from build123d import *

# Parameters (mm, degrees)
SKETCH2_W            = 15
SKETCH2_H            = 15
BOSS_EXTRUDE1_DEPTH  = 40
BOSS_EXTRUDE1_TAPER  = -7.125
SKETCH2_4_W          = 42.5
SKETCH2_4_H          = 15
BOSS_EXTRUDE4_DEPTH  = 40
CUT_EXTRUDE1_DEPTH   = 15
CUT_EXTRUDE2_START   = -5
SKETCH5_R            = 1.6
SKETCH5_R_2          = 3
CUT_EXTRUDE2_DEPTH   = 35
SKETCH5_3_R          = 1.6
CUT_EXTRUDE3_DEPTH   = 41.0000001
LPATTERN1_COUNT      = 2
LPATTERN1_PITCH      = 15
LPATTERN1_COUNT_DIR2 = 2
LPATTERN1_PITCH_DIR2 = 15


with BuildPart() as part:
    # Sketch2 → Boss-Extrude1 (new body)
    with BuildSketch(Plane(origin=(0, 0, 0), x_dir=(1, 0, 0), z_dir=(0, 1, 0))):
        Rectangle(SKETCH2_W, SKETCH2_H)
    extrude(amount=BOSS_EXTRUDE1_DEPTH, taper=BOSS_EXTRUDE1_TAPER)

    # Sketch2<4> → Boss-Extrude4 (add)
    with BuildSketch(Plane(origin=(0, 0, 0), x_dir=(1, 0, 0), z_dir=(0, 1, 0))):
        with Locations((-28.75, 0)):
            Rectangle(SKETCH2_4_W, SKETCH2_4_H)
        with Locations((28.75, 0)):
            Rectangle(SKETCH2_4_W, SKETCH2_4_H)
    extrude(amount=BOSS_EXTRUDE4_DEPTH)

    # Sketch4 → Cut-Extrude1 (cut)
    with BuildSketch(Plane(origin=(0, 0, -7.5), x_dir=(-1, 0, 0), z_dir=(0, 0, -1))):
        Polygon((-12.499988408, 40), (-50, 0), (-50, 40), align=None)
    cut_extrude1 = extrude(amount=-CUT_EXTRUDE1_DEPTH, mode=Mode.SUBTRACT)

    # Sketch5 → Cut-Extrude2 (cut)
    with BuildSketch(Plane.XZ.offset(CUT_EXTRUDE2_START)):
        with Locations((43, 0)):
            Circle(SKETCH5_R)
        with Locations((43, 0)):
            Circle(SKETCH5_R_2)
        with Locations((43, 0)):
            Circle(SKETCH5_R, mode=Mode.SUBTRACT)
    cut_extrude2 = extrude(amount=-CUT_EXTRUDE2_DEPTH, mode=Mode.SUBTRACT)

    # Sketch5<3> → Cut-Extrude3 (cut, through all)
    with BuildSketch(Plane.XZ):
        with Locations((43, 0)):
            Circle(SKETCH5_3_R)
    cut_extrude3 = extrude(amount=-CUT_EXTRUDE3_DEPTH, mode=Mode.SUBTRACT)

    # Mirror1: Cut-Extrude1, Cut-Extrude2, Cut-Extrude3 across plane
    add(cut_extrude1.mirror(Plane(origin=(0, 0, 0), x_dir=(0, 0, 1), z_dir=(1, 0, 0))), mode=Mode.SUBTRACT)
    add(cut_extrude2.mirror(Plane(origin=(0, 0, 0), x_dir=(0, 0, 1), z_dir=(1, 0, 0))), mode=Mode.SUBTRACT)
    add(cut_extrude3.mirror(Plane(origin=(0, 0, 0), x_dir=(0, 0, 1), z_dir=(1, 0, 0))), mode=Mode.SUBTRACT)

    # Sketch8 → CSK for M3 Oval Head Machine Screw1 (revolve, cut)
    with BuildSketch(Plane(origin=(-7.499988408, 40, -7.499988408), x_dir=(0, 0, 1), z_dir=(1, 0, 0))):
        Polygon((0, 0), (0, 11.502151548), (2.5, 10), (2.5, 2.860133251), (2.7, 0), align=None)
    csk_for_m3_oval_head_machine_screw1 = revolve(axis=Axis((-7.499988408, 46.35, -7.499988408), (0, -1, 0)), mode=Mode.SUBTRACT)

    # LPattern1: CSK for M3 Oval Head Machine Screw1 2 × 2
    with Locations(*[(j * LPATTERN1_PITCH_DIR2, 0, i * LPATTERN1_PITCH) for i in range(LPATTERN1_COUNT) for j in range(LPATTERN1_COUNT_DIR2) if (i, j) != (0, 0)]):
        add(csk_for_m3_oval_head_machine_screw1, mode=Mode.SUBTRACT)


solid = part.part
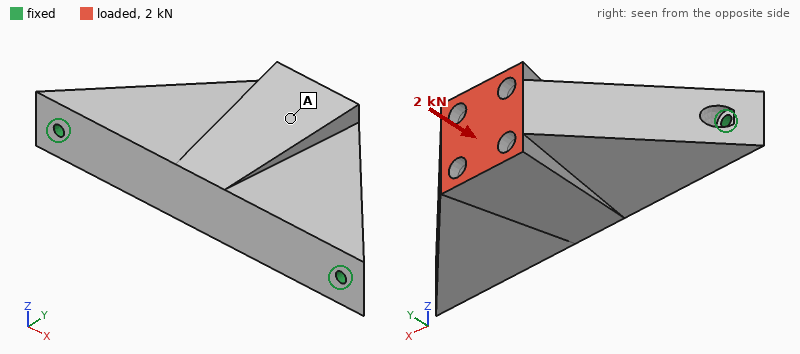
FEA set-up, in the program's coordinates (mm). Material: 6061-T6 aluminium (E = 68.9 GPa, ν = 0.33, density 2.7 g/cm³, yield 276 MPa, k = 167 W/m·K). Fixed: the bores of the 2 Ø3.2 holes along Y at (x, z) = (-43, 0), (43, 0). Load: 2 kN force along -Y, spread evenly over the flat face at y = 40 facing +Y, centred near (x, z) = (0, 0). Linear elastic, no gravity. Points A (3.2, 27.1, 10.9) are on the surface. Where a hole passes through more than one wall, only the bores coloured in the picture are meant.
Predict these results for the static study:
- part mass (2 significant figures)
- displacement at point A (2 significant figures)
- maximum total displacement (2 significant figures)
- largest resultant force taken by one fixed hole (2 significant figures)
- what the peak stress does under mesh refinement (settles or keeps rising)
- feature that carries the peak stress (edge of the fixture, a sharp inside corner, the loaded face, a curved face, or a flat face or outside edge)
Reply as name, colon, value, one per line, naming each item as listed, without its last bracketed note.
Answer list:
part mass: 110 g
displacement at point A: 11 µm
maximum total displacement: 12 µm
largest resultant force taken by one fixed hole: 1.3 kN
what the peak stress does under mesh refinement: keeps rising
feature that carries the peak stress: edge of the fixture
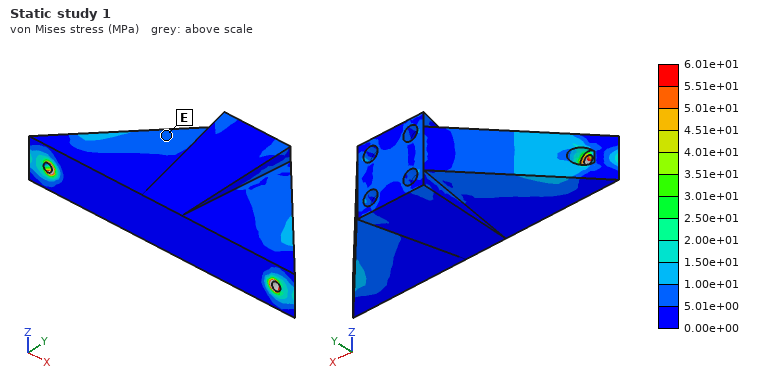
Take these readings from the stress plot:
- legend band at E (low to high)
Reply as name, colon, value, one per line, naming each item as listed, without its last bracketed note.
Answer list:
legend band at E: 5.01e+00 to 1.00e+01 MPa
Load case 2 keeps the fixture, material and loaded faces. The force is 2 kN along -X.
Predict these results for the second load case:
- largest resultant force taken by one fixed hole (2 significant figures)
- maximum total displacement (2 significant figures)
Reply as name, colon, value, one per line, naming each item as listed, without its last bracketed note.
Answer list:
largest resultant force taken by one fixed hole: 1.3 kN
maximum total displacement: 11 µm
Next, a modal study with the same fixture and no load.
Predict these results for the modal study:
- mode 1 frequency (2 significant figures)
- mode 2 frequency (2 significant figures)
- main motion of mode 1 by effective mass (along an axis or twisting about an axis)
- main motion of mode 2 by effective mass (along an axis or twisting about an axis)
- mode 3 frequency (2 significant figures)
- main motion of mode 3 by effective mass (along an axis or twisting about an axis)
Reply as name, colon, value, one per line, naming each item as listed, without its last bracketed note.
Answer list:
mode 1 frequency: 1900 Hz
mode 2 frequency: 7000 Hz
main motion of mode 1 by effective mass: along Z
main motion of mode 2 by effective mass: along Z
mode 3 frequency: 7400 Hz
main motion of mode 3 by effective mass: along Y
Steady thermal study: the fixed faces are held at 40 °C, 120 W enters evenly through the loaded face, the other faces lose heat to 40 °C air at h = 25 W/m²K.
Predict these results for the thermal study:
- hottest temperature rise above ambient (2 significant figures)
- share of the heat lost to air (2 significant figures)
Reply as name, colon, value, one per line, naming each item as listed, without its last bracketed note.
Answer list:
hottest temperature rise above ambient: 80 K
share of the heat lost to air: 9.2 %
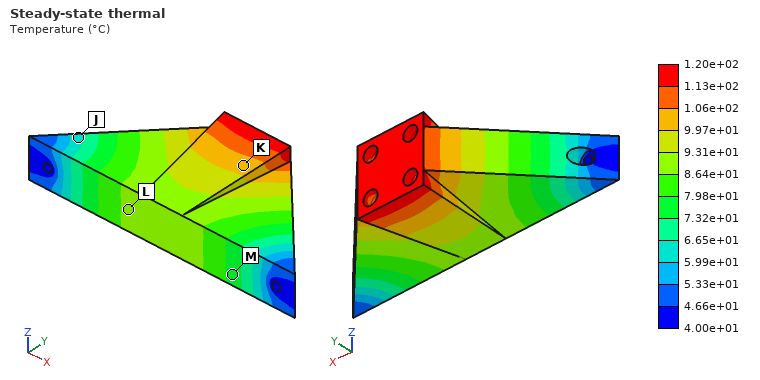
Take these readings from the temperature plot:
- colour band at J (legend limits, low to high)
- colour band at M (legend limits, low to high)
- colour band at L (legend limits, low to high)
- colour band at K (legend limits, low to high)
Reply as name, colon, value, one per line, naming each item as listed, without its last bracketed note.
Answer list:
colour band at J: 5.99e+01 to 6.65e+01 °C
colour band at M: 7.32e+01 to 7.98e+01 °C
colour band at L: 8.64e+01 to 9.31e+01 °C
colour band at K: 9.97e+01 to 1.06e+02 °C
